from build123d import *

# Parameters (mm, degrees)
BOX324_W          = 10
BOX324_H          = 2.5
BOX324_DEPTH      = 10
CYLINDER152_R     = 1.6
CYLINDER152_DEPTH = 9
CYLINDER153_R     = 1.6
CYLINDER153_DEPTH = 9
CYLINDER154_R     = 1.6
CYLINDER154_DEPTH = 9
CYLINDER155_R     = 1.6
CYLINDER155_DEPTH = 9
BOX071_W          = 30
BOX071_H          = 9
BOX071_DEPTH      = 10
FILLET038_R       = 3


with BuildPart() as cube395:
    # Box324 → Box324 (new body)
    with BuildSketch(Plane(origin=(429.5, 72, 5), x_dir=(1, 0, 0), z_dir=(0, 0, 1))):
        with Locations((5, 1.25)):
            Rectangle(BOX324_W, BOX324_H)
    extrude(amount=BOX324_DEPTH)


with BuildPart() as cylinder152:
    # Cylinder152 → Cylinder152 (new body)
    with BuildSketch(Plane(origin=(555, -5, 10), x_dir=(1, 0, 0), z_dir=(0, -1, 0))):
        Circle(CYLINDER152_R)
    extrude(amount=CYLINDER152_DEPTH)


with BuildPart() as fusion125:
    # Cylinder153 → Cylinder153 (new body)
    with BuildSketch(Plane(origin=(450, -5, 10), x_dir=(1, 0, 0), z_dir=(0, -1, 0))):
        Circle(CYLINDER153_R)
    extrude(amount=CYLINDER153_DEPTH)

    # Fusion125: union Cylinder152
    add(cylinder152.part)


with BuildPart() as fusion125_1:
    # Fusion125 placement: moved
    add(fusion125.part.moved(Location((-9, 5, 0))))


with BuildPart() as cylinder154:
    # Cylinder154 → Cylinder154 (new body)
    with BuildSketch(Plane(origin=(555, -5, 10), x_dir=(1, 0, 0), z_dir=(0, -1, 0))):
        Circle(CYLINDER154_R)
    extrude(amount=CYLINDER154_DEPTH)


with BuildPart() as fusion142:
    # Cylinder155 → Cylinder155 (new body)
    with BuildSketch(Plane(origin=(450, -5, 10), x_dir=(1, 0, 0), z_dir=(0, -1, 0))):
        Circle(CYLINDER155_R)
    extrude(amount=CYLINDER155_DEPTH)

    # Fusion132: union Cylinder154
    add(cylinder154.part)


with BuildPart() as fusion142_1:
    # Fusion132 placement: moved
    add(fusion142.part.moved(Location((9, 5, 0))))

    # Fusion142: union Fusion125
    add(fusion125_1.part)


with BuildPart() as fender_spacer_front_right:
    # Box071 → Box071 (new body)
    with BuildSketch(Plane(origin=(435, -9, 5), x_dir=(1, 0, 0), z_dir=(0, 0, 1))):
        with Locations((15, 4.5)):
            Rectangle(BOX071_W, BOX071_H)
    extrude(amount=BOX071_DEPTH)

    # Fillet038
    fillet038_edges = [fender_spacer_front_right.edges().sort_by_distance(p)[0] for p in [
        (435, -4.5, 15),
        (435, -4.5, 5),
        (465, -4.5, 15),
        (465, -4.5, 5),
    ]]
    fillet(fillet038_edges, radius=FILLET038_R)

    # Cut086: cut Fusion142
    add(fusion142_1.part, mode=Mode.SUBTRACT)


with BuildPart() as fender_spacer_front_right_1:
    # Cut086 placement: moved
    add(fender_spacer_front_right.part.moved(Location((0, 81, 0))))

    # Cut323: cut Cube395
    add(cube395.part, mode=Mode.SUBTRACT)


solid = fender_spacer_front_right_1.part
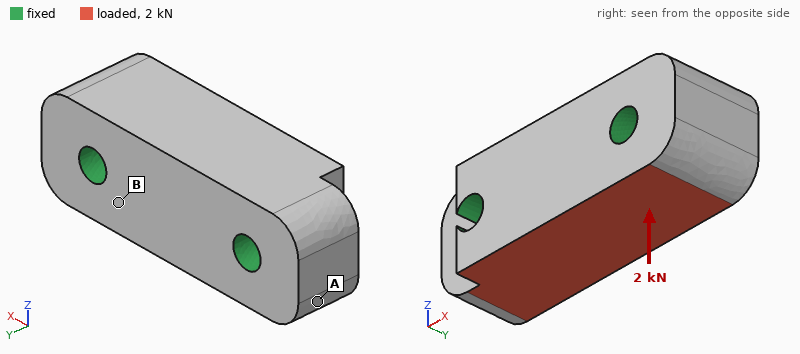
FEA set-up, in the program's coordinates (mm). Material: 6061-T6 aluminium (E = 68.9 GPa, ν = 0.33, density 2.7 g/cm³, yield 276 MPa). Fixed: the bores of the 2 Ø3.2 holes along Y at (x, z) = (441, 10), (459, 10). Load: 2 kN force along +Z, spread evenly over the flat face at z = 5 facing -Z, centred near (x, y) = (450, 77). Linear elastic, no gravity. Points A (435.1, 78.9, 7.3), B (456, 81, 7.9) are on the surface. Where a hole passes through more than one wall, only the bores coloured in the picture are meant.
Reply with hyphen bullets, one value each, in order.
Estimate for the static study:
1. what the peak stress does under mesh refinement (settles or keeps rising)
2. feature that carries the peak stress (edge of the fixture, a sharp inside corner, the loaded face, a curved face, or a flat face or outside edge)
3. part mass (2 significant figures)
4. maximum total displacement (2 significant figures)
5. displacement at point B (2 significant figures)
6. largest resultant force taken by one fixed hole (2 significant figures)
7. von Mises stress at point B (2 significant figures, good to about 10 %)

- keeps rising
- edge of the fixture
- 6.4 g
- 2.7 µm
- 1.1 µm
- 1.0 kN
- 15 MPa
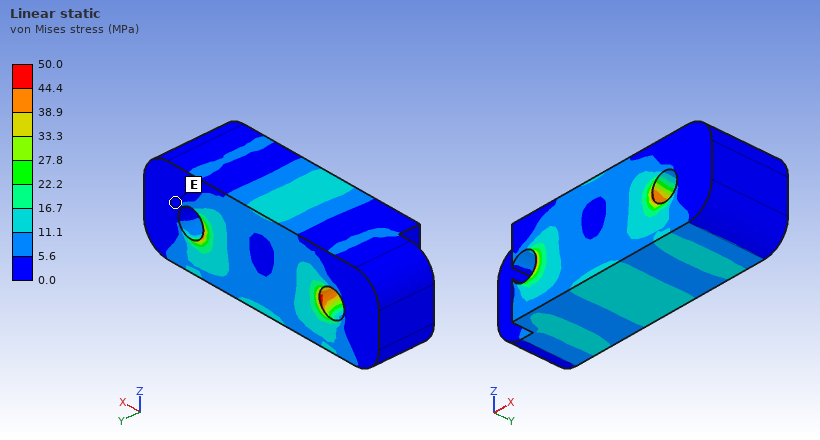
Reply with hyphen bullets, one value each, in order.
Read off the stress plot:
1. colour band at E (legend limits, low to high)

- 0.0 to 5.6 MPa
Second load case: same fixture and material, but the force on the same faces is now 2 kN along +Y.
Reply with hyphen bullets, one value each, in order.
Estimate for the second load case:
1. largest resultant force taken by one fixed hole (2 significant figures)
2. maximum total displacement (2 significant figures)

- 1.0 kN
- 7.5 µm
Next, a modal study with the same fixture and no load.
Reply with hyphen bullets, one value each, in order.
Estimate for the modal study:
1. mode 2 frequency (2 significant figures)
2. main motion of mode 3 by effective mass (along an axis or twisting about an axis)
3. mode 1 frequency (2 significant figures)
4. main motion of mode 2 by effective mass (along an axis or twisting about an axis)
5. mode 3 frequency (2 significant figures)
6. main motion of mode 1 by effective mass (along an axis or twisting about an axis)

- 72 kHz
- twisting about X
- 66 kHz
- along Y
- 79 kHz
- along Z
